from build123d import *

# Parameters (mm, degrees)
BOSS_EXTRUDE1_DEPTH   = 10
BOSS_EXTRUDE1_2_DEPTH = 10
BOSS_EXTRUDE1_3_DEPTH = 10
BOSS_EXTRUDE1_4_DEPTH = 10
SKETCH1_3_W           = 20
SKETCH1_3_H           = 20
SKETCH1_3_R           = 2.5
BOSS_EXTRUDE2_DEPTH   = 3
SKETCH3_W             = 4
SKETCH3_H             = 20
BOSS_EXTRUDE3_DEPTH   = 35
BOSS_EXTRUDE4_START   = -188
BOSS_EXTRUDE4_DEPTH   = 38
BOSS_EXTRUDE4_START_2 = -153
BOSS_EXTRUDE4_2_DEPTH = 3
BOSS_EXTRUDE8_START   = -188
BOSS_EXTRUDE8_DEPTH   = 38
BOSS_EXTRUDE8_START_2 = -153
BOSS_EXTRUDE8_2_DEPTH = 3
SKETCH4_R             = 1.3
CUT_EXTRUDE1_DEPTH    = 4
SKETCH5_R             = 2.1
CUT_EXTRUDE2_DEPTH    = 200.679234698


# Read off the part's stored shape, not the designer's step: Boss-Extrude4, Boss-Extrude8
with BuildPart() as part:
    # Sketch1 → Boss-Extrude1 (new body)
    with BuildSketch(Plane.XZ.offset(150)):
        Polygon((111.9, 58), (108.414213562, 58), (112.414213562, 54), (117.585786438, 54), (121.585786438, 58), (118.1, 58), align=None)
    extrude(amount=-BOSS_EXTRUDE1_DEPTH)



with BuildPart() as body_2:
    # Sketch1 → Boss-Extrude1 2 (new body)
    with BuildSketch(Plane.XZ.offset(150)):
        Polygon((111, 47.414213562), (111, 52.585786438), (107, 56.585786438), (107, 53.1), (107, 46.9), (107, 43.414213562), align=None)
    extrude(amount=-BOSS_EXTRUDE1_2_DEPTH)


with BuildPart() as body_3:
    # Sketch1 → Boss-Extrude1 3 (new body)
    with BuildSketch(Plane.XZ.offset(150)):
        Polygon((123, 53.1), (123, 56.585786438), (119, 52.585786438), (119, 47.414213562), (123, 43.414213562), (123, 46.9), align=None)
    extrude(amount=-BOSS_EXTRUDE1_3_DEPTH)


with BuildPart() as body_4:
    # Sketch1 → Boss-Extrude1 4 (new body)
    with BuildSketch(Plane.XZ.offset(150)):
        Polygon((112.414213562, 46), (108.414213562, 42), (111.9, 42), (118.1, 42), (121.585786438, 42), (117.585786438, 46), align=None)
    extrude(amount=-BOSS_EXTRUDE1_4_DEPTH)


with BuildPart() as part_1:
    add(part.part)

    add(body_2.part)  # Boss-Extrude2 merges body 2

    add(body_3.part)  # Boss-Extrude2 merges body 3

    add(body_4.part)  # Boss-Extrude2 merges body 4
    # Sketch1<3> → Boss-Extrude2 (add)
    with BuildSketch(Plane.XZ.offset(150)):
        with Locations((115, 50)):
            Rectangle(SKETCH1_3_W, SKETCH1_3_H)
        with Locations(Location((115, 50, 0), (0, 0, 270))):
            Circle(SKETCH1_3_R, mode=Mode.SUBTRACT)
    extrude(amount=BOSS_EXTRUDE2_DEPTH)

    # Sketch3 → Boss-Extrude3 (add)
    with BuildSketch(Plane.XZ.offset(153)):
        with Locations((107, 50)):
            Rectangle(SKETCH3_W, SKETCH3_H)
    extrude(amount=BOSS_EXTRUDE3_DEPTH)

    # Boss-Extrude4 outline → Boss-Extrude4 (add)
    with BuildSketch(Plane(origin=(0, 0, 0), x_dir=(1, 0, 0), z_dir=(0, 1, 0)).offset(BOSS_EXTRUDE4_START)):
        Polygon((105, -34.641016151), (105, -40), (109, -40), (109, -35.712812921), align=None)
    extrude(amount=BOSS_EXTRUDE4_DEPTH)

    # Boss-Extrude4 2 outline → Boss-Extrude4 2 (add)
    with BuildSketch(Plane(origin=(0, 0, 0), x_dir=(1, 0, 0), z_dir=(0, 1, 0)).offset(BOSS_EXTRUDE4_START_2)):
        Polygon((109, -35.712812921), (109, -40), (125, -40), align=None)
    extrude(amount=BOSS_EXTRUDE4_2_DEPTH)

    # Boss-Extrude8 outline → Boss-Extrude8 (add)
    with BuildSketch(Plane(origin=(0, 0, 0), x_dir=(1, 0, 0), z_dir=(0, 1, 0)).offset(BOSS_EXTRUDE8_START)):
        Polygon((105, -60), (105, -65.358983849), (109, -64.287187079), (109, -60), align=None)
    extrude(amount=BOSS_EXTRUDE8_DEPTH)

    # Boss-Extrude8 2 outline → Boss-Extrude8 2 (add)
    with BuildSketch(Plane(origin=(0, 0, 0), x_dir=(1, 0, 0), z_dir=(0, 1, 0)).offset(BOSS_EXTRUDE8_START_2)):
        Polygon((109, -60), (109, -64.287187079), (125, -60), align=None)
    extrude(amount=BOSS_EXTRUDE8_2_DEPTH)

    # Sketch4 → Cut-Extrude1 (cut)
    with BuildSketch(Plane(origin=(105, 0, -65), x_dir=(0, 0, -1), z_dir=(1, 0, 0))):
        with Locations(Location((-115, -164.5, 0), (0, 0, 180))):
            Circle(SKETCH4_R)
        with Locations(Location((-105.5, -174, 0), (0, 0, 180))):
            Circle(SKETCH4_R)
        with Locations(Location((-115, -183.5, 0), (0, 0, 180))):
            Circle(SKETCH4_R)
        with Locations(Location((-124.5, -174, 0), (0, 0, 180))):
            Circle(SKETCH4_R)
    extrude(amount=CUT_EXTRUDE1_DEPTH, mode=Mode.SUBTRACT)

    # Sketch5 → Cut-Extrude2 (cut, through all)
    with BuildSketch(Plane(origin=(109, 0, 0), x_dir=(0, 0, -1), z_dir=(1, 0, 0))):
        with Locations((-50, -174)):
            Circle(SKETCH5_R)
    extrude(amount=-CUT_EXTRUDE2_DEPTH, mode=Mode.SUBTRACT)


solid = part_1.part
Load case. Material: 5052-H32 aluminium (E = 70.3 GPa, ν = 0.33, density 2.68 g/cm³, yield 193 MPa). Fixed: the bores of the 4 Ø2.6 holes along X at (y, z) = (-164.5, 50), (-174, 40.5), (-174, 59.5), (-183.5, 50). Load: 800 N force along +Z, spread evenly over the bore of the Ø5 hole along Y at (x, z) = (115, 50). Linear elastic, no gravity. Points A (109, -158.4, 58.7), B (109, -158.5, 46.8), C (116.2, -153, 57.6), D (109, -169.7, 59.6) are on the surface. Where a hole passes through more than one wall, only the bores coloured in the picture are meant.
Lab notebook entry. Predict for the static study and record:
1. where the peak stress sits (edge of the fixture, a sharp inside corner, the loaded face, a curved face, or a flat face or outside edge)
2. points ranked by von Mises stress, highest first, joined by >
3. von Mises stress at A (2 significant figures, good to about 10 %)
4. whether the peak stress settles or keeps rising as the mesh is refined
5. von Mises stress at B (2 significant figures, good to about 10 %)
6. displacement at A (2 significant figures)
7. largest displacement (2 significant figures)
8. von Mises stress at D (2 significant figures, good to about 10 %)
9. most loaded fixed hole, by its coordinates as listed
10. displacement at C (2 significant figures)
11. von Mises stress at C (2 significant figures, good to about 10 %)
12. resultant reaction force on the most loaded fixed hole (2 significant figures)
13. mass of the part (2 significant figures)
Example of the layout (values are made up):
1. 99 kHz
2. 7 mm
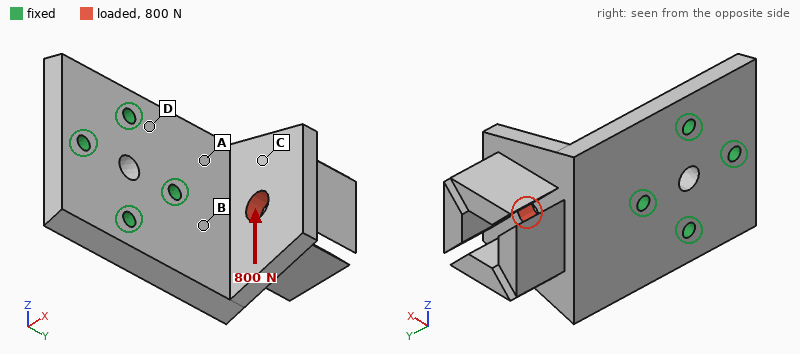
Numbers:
1. edge of the fixture
2. B > A > D > C
3. 56 MPa
4. keeps rising
5. 68 MPa
6. 0.027 mm
7. 0.11 mm
8. 35 MPa
9. (-164.5, 50)
10. 0.065 mm
11. 19 MPa
12. 850 N
13. 19 g
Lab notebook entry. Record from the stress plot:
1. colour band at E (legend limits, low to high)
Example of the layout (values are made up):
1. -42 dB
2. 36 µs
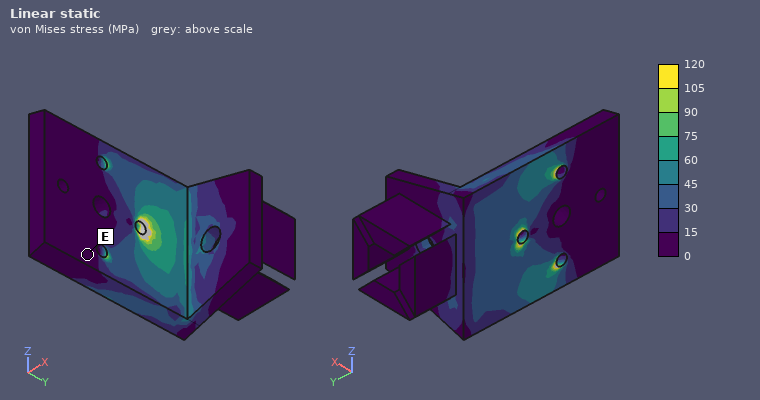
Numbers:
1. 0 to 15 MPa
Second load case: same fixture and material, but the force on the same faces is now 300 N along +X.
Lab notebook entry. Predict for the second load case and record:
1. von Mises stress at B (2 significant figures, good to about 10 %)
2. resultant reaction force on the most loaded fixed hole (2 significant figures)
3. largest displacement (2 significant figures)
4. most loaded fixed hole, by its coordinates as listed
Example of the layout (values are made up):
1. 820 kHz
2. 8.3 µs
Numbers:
1. 28 MPa
2. 450 N
3. 76 µm
4. (-164.5, 50)
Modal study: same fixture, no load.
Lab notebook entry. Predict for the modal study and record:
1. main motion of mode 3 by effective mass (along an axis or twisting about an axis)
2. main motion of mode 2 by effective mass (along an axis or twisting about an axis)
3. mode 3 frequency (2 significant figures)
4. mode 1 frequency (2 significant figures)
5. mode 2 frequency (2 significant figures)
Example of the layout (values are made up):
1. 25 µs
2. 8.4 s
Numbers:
1. along X
2. along Z
3. 9600 Hz
4. 3100 Hz
5. 5500 Hz
